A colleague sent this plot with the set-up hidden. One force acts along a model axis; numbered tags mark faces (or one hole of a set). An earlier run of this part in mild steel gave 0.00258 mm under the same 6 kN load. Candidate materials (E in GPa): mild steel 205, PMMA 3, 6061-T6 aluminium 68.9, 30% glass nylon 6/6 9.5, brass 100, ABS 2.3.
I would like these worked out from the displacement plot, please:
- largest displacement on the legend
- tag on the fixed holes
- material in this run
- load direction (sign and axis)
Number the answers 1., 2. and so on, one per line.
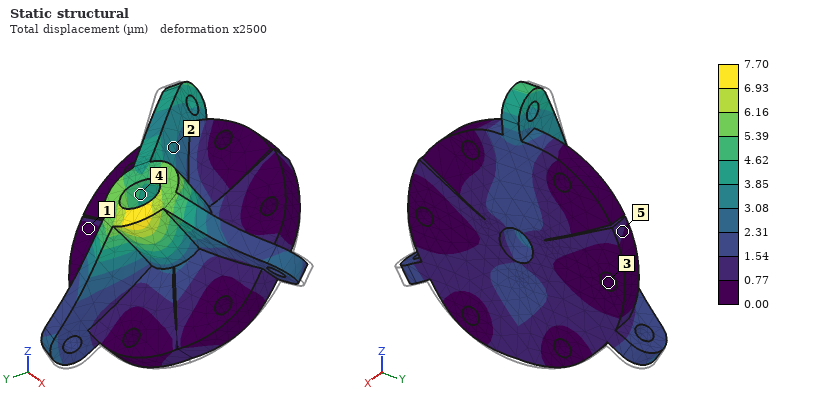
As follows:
1. 7.70 µm
2. 3
3. 6061-T6 aluminium
4. +Z
